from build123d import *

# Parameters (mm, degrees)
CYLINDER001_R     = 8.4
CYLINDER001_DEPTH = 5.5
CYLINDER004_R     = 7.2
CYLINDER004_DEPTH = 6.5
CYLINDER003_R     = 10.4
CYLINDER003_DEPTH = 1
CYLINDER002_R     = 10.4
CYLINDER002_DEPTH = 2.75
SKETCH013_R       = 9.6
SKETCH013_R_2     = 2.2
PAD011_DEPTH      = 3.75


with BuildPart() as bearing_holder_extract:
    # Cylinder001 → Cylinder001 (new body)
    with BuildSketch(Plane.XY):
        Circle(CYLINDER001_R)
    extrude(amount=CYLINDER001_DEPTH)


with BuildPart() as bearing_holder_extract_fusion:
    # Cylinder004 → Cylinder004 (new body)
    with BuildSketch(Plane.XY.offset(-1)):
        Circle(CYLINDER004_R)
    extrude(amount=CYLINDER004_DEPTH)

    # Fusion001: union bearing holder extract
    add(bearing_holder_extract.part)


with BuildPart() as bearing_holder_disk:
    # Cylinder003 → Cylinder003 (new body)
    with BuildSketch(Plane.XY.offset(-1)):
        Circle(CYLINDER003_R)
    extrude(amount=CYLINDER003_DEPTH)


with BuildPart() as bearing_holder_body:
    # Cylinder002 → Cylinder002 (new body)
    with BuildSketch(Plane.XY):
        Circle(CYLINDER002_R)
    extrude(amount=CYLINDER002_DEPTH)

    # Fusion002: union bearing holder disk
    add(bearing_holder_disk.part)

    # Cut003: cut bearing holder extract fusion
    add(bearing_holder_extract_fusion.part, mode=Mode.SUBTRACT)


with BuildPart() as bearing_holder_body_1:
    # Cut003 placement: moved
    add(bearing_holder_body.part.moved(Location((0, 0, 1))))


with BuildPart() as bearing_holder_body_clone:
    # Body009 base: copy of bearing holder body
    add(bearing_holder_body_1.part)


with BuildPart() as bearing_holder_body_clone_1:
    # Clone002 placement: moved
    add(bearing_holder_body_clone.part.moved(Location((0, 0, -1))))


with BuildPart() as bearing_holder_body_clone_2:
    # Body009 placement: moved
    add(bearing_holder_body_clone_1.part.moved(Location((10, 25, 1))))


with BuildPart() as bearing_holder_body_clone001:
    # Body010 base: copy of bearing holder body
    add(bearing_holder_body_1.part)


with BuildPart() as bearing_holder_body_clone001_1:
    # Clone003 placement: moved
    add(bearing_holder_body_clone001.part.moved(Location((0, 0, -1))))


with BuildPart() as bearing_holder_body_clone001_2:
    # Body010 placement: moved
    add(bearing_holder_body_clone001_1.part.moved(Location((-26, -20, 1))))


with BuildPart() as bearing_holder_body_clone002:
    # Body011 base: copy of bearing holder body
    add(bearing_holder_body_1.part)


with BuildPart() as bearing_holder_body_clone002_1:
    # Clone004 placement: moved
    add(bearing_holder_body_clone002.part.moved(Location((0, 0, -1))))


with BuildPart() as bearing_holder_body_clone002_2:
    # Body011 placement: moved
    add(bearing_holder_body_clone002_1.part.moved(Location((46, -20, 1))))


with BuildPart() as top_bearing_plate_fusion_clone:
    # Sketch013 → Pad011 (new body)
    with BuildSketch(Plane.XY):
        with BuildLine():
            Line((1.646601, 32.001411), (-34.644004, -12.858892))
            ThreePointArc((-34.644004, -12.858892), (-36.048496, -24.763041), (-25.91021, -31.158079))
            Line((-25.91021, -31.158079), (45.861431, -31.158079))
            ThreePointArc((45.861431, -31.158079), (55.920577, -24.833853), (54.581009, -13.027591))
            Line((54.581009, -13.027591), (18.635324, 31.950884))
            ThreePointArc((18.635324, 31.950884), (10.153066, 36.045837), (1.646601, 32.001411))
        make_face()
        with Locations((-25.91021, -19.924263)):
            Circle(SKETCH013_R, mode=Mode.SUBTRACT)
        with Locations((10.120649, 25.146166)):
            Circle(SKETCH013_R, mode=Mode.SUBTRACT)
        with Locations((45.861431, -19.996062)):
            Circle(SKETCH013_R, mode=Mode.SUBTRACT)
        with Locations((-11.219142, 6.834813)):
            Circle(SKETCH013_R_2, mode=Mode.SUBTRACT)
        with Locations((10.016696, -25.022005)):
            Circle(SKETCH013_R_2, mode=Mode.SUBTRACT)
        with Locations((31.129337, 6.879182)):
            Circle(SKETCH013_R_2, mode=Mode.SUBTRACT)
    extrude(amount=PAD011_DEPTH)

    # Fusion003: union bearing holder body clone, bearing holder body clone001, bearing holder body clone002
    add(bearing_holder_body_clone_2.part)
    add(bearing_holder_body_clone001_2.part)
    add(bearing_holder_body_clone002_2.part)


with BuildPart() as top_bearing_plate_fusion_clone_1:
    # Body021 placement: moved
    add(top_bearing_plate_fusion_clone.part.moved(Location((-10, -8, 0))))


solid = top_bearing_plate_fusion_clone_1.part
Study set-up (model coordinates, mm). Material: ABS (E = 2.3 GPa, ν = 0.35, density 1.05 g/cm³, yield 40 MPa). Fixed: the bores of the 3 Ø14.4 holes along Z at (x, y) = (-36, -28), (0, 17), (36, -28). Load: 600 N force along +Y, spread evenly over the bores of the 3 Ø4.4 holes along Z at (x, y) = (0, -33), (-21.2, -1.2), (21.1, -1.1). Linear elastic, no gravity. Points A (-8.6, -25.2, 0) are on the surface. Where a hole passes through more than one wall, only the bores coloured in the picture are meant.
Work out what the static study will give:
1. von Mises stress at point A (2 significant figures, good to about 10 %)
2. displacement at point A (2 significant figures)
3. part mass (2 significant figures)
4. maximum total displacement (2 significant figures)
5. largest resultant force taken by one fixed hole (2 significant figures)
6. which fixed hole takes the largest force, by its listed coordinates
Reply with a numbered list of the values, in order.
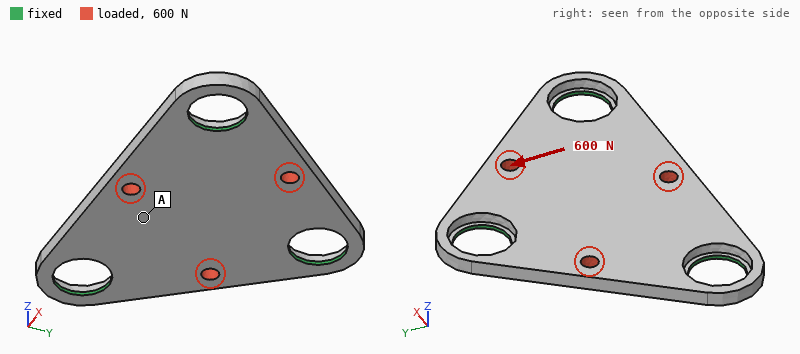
1. 1.7 MPa
2. 48 µm
3. 13 g
4. 77 µm
5. 290 N
6. (0, 17)
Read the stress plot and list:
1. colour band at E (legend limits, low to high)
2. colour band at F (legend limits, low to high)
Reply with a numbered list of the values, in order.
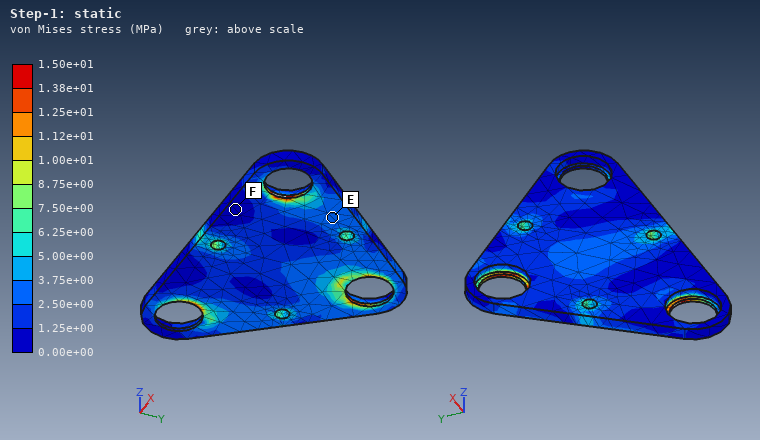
1. 2.50e+00 to 3.75e+00 MPa
2. 0.00e+00 to 1.25e+00 MPa
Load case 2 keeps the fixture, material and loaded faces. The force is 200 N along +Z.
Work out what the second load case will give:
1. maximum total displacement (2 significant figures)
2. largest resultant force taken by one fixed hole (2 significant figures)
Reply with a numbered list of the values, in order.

1. 0.60 mm
2. 160 N
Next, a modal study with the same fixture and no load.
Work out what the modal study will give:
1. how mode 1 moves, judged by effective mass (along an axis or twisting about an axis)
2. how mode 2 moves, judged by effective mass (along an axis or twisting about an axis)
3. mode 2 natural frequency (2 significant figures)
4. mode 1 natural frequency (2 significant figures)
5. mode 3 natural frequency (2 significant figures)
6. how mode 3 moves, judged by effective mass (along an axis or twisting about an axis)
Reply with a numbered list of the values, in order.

1. along Z
2. along Z
3. 2000 Hz
4. 1300 Hz
5. 2100 Hz
6. twisting about Y
